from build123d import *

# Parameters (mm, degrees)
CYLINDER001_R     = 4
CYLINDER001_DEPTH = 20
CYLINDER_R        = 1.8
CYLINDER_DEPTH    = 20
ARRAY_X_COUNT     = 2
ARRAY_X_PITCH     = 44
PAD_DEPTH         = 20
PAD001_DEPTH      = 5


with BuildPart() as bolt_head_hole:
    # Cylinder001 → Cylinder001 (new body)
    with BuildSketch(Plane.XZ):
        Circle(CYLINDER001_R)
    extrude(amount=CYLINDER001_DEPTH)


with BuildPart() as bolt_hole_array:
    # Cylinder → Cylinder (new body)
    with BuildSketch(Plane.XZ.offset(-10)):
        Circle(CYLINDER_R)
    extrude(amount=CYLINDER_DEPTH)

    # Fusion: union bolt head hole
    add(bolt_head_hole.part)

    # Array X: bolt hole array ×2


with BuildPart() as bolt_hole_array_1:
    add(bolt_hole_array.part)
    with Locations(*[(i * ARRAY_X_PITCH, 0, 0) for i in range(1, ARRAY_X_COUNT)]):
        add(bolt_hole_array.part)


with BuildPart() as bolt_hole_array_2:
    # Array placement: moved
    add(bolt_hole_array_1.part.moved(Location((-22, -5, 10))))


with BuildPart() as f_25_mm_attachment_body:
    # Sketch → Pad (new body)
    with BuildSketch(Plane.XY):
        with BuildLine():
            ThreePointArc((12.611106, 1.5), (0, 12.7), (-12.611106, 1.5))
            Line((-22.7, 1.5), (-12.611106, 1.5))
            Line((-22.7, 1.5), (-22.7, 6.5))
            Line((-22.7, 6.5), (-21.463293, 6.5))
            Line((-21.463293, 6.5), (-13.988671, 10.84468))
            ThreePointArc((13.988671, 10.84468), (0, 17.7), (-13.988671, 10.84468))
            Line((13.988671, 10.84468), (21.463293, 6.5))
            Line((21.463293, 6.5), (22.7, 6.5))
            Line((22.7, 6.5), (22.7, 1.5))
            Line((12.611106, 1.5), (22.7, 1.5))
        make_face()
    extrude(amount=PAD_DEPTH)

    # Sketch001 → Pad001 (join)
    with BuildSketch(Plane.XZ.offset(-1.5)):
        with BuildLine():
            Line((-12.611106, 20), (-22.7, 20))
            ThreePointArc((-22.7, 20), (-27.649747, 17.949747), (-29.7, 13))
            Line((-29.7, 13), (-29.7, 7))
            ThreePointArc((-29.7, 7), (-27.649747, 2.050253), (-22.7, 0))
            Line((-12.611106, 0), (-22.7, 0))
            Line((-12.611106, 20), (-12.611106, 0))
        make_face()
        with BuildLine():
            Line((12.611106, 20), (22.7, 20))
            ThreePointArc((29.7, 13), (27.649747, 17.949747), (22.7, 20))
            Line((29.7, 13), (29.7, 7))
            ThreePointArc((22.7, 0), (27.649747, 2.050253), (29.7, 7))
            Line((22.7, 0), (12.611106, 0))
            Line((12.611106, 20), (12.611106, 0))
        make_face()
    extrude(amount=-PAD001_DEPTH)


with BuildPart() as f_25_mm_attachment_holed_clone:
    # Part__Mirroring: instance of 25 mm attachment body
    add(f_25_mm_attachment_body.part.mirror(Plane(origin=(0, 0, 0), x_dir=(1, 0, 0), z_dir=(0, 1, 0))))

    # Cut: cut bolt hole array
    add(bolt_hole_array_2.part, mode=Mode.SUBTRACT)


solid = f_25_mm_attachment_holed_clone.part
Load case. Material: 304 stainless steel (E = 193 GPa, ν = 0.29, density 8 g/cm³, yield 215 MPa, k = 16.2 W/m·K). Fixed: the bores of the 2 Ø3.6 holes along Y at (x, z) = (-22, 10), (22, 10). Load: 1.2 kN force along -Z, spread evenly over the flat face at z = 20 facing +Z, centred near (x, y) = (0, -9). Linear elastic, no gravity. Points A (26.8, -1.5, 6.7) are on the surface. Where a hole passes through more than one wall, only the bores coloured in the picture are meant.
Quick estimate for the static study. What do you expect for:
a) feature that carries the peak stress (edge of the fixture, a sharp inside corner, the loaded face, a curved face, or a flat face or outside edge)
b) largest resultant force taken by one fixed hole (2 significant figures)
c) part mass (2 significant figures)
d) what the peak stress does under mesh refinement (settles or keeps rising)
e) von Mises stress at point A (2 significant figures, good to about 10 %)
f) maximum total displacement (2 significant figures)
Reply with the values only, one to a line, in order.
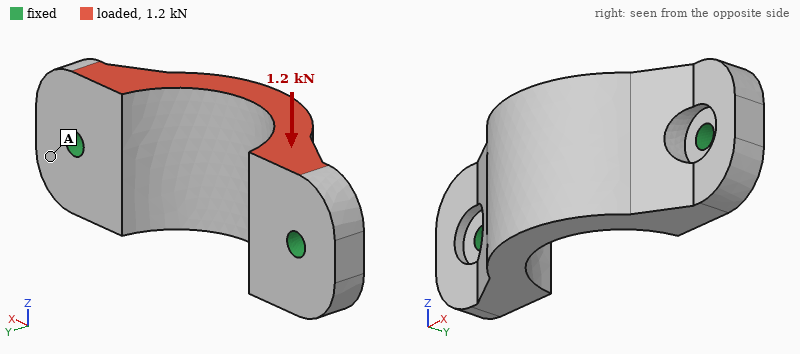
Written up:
edge of the fixture
600 N
55 g
keeps rising
19 MPa
18 µm
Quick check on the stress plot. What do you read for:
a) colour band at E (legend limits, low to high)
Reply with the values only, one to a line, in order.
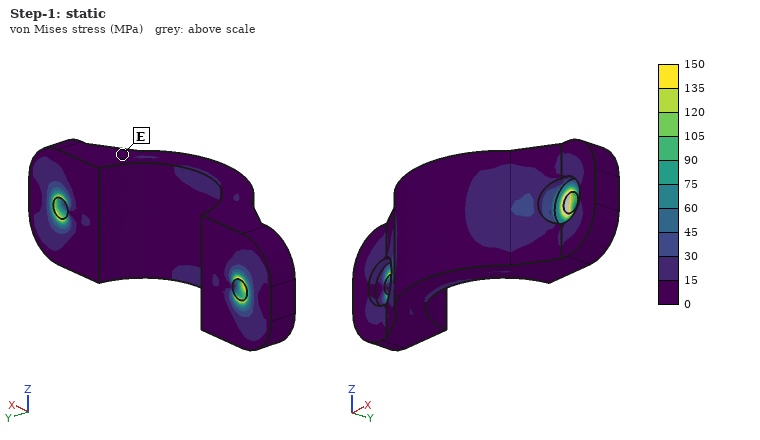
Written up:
0 to 15 MPa
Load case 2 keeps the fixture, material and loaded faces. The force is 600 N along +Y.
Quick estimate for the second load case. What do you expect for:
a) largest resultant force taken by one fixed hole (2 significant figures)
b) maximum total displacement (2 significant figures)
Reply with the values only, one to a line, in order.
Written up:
370 N
12 µm
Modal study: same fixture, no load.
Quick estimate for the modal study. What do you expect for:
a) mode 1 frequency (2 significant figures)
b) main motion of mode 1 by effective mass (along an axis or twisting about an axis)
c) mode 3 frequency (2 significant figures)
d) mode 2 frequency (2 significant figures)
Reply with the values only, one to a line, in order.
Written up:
7100 Hz
along Z
18 kHz
18 kHz
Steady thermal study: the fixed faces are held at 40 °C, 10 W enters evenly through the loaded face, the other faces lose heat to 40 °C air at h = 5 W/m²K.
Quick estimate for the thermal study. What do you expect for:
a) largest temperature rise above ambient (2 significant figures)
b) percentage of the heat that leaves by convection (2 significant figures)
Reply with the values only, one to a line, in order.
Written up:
56 K
4.3 %
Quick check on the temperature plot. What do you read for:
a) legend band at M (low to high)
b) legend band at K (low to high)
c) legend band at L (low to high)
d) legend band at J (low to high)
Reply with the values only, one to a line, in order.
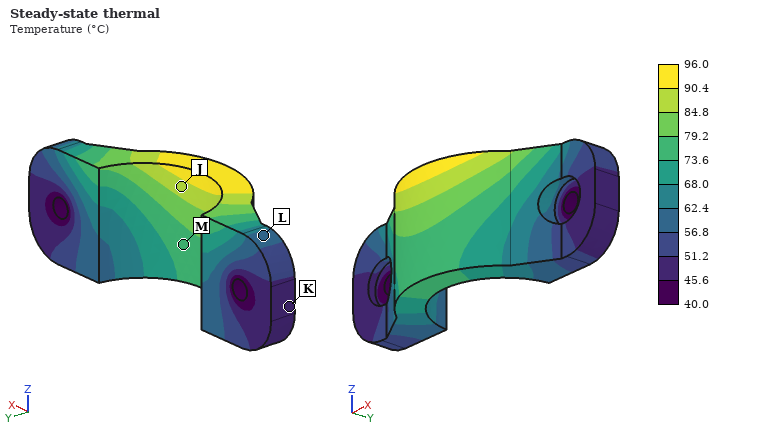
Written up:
73.6 to 79.2 °C
45.6 to 51.2 °C
56.8 to 62.4 °C
84.8 to 90.4 °C
